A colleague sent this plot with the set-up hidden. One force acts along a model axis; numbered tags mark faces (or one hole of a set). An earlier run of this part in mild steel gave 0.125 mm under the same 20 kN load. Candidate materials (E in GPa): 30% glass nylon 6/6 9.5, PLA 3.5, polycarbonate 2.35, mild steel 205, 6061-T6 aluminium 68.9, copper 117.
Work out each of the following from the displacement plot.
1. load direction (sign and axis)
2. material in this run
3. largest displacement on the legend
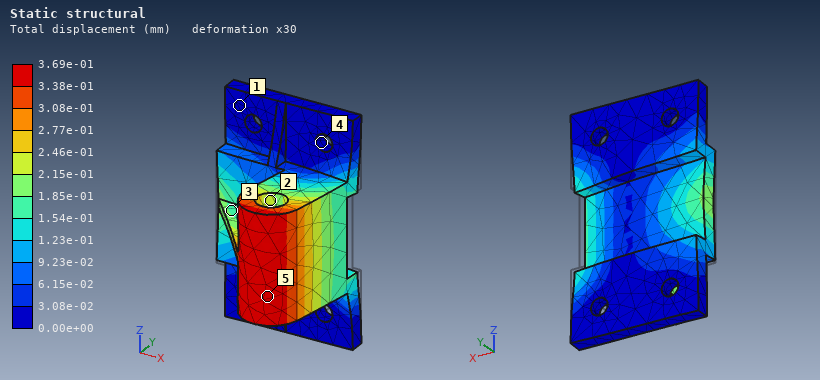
-X
6061-T6 aluminium
3.69e-01 mm
